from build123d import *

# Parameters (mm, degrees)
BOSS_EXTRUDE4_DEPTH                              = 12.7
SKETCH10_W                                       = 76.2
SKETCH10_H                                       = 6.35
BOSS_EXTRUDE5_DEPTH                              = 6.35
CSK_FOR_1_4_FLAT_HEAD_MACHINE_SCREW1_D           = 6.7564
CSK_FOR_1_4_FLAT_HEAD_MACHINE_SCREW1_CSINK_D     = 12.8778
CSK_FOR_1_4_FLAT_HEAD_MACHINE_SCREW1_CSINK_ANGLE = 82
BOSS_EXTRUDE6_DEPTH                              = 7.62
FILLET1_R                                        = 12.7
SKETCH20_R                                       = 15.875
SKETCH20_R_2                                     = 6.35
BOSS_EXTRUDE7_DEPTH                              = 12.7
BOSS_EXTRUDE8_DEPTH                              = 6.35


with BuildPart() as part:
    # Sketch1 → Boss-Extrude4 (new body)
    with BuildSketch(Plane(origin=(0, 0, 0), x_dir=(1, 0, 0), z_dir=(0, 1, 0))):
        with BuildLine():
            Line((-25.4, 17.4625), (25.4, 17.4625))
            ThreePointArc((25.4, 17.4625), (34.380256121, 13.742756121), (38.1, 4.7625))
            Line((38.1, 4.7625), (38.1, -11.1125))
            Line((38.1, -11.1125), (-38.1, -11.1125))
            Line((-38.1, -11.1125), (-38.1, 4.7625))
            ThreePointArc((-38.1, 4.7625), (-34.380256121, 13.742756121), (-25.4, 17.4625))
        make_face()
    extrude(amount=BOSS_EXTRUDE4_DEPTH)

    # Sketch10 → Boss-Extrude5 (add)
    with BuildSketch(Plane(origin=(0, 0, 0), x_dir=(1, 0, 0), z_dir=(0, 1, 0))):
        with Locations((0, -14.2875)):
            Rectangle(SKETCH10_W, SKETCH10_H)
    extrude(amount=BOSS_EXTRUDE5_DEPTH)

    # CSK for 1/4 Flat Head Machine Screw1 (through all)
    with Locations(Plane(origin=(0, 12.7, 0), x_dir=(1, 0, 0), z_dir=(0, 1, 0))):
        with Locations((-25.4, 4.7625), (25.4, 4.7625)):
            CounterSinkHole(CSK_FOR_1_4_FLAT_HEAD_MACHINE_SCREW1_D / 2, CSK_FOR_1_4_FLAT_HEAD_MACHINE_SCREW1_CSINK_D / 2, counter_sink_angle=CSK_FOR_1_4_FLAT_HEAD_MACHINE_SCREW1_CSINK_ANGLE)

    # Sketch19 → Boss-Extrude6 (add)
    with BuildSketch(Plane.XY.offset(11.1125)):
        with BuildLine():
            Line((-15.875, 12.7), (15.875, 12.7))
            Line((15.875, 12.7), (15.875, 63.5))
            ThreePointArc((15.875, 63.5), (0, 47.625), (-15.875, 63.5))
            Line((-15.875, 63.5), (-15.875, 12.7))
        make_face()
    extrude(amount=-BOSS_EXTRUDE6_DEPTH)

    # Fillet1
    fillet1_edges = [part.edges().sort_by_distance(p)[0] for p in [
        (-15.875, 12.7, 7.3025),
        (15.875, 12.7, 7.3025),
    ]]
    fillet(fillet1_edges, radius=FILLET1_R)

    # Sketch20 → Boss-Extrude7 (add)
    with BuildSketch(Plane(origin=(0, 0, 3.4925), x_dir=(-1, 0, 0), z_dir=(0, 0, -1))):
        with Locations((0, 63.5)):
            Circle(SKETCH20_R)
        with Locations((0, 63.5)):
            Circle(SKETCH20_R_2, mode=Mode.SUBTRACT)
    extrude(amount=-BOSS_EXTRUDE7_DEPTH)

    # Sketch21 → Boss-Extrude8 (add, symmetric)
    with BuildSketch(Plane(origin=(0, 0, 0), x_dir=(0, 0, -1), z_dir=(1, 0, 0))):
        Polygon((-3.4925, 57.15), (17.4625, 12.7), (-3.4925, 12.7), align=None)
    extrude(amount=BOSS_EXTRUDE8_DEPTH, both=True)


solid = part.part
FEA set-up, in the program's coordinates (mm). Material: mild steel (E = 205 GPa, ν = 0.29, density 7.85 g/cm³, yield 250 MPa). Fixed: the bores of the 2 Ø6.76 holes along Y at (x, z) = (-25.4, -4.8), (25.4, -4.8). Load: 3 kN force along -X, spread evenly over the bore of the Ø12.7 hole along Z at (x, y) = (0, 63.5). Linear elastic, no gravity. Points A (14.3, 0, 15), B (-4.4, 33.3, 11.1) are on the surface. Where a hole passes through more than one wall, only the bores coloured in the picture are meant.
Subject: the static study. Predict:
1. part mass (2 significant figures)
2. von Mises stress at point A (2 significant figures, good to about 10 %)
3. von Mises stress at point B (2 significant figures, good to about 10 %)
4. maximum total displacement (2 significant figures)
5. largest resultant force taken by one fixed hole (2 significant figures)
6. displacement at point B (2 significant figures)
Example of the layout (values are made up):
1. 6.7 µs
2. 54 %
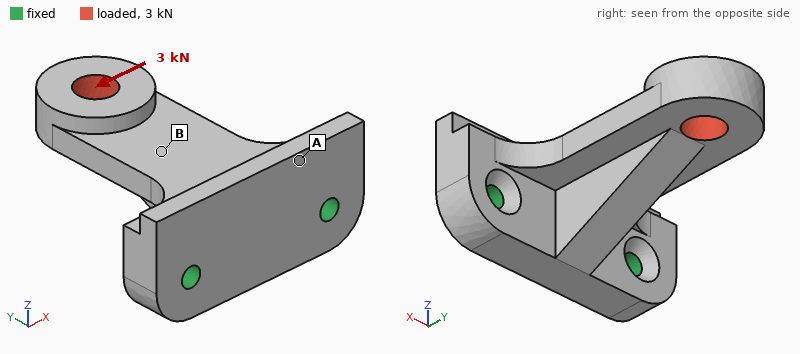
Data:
1. 410 g
2. 22 MPa
3. 47 MPa
4. 69 µm
5. 4.1 kN
6. 14 µm
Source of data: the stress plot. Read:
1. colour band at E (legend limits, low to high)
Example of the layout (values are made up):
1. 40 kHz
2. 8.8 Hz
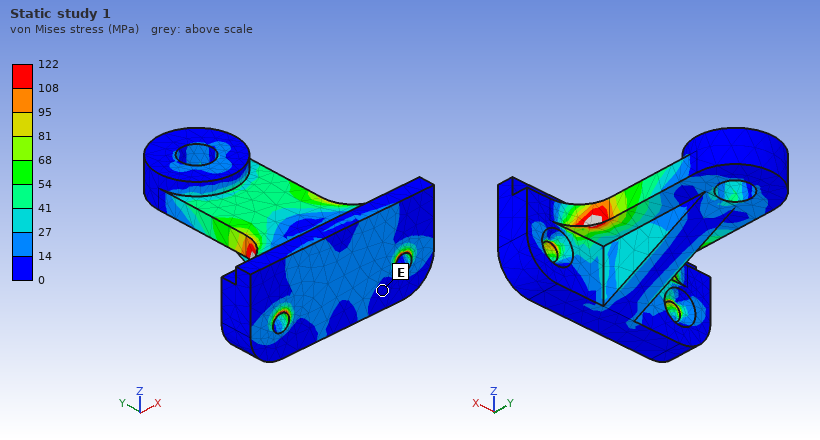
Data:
1. 0 to 14 MPa
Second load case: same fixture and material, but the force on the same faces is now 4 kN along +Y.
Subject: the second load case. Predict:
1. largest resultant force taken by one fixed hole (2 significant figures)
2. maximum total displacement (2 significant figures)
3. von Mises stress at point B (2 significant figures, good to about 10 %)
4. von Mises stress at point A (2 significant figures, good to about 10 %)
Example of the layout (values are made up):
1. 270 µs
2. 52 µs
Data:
1. 2.1 kN
2. 58 µm
3. 27 MPa
4. 12 MPa
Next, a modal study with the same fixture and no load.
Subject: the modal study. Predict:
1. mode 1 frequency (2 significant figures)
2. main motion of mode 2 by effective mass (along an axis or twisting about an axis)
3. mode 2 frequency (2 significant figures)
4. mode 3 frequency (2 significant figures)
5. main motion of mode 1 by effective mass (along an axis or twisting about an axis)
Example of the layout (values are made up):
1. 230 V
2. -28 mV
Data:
1. 2300 Hz
2. along X
3. 4300 Hz
4. 7900 Hz
5. along Z
